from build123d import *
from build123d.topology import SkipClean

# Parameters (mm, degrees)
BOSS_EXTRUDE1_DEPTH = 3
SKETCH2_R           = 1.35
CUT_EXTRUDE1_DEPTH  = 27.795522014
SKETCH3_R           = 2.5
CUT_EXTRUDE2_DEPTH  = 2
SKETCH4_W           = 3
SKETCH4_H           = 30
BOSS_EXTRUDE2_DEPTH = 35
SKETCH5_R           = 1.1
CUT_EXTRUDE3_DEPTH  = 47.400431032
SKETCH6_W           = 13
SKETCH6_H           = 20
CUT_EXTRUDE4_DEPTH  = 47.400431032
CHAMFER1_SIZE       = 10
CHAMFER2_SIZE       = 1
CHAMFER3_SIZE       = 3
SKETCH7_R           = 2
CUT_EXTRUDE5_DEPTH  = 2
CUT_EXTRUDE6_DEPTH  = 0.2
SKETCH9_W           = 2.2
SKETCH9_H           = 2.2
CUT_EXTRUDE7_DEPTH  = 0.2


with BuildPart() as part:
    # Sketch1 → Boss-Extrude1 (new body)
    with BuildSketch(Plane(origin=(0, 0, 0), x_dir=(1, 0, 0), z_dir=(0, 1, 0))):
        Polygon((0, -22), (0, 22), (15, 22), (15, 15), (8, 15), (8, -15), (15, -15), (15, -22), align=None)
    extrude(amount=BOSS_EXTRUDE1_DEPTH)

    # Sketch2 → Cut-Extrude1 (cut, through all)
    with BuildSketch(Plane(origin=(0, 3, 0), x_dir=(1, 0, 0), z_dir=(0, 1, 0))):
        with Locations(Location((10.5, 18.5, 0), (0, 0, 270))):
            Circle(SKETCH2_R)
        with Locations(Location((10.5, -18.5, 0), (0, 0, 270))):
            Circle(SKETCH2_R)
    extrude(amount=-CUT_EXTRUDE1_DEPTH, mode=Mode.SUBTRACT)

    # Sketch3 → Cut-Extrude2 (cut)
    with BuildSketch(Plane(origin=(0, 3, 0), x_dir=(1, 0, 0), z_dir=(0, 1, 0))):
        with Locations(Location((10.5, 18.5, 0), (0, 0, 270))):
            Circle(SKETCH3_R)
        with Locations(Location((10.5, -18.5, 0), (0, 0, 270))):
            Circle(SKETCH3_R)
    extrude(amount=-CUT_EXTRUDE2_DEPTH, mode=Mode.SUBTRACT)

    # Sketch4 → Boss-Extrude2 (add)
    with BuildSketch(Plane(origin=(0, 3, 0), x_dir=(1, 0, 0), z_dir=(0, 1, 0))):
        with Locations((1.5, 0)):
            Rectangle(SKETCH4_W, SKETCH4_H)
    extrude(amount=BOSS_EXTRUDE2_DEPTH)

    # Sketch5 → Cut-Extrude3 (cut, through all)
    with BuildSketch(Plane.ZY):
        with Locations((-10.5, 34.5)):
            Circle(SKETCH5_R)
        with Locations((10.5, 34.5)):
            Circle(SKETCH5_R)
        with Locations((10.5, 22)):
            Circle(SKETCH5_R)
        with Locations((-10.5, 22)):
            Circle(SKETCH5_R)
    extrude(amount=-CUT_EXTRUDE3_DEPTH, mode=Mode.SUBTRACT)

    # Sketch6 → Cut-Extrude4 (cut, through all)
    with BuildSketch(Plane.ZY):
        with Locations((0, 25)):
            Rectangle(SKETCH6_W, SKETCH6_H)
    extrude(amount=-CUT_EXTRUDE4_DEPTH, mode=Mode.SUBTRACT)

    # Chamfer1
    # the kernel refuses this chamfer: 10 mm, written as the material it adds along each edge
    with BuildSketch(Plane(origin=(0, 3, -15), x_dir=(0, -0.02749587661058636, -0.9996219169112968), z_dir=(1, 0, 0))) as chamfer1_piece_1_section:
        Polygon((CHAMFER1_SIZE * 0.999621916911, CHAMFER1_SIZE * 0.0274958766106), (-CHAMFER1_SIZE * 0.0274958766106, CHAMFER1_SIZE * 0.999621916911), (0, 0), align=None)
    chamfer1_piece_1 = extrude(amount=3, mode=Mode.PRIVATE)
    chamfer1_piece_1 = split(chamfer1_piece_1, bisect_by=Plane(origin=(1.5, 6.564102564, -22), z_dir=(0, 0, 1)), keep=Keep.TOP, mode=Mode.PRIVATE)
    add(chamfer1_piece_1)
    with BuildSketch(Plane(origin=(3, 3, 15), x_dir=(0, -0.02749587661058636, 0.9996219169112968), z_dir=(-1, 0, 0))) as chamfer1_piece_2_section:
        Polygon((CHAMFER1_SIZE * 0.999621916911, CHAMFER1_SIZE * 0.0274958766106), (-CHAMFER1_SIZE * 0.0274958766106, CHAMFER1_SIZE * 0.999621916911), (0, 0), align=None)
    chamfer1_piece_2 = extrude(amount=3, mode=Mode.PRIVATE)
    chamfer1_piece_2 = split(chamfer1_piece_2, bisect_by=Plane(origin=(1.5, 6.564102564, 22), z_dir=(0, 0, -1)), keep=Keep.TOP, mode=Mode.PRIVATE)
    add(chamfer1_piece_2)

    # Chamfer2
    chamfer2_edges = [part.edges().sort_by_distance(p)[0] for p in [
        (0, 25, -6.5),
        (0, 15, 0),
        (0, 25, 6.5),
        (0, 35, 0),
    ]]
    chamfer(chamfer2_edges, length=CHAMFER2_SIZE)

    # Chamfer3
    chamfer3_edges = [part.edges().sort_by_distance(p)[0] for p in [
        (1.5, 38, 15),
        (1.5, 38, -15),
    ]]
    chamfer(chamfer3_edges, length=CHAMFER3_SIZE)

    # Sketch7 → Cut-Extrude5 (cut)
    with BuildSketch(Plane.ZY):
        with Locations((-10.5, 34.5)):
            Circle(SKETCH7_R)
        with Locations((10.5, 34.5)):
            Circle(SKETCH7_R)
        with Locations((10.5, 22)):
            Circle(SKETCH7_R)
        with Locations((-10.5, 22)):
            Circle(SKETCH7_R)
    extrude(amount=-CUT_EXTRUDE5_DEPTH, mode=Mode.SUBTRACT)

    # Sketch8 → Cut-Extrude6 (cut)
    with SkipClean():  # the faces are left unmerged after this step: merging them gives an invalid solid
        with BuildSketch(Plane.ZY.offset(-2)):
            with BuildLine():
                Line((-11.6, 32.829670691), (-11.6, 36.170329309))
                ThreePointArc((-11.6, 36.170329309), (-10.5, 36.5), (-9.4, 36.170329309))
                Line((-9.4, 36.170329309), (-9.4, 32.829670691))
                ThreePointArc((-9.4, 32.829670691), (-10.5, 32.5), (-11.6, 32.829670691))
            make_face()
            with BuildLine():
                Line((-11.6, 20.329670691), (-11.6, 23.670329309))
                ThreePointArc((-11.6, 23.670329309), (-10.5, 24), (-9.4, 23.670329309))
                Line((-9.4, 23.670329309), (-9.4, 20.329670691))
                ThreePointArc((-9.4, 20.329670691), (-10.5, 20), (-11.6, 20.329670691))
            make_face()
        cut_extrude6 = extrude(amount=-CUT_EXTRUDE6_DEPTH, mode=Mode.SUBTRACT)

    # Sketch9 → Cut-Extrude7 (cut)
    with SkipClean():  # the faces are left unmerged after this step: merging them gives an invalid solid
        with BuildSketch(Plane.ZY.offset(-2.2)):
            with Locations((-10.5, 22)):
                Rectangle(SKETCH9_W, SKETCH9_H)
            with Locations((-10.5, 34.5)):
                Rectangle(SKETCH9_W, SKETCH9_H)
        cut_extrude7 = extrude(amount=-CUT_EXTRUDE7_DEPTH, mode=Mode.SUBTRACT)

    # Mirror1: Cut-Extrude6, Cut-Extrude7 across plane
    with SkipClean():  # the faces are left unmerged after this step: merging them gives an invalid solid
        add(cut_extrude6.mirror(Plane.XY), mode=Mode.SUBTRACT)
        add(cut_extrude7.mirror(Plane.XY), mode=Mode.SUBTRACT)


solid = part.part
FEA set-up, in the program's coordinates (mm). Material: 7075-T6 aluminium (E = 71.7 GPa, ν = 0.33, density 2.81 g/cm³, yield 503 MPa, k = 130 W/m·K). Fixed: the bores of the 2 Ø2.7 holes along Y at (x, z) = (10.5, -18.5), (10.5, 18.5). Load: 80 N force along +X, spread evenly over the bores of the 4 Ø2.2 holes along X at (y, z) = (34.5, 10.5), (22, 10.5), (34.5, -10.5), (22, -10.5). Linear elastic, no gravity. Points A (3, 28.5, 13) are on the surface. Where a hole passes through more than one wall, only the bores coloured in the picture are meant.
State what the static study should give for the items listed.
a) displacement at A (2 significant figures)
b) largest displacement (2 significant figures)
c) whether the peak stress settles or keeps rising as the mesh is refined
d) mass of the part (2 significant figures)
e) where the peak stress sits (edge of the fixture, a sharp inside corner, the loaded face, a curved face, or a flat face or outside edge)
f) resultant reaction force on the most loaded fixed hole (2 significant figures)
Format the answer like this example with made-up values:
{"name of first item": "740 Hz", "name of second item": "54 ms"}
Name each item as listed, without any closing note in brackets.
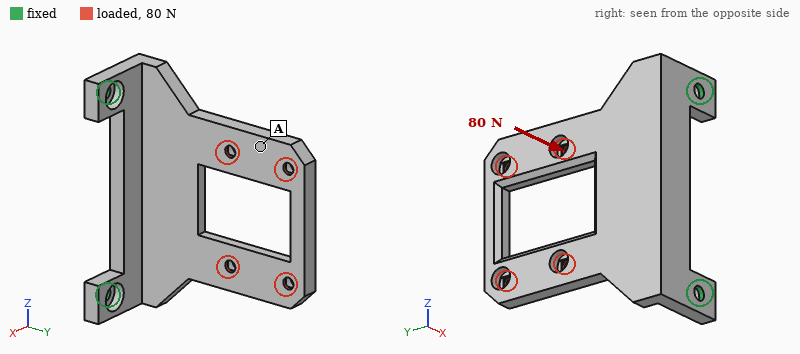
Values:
{"displacement at A": "0.49 mm", "largest displacement": "0.71 mm", "whether the peak stress settles or keeps rising as the mesh is refined": "keeps rising", "mass of the part": "10 g", "where the peak stress sits": "edge of the fixture", "resultant reaction force on the most loaded fixed hole": "58 N"}
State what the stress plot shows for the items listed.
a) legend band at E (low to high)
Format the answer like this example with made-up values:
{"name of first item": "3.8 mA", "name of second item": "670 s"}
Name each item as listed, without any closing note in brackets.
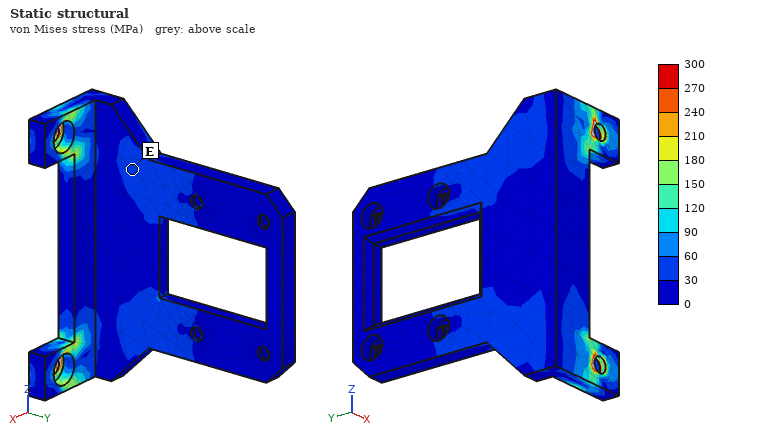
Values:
{"legend band at E": "30 to 60 MPa"}
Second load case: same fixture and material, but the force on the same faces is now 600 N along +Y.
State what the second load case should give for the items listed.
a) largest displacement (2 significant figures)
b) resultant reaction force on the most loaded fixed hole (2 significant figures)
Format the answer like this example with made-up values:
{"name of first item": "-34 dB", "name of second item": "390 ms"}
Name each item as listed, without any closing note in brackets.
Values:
{"largest displacement": "0.65 mm", "resultant reaction force on the most loaded fixed hole": "300 N"}
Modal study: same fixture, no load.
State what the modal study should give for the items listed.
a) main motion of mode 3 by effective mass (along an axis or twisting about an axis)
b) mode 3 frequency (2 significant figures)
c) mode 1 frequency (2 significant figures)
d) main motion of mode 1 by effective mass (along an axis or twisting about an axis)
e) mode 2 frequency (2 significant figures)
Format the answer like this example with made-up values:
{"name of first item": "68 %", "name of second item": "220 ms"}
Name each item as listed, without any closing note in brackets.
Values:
{"main motion of mode 3 by effective mass": "along Y", "mode 3 frequency": "4600 Hz", "mode 1 frequency": "1100 Hz", "main motion of mode 1 by effective mass": "along X", "mode 2 frequency": "3700 Hz"}
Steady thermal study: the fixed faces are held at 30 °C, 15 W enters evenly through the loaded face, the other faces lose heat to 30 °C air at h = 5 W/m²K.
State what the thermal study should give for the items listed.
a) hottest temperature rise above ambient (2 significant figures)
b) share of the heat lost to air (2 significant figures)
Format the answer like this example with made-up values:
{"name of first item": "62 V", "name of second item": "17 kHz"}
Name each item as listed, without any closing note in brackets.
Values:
{"hottest temperature rise above ambient": "85 K", "share of the heat lost to air": "4.8 %"}
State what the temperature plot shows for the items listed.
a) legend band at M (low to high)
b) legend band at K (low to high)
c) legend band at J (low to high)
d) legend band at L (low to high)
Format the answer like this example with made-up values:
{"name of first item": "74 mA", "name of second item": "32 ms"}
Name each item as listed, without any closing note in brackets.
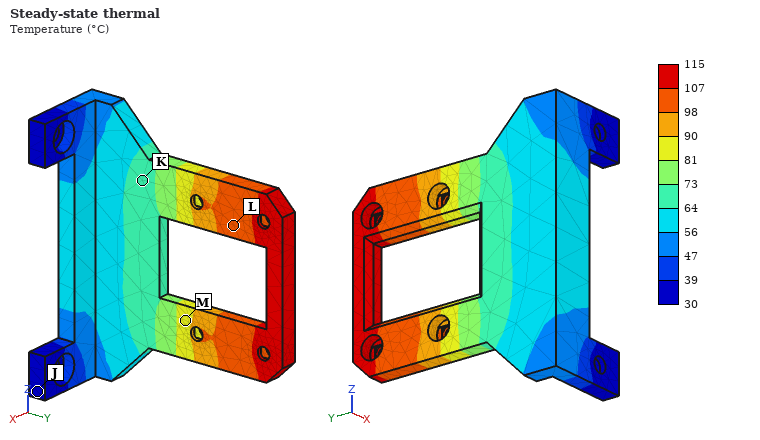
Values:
{"legend band at M": "81 to 90 °C", "legend band at K": "64 to 73 °C", "legend band at J": "30 to 39 °C", "legend band at L": "98 to 107 °C"}
